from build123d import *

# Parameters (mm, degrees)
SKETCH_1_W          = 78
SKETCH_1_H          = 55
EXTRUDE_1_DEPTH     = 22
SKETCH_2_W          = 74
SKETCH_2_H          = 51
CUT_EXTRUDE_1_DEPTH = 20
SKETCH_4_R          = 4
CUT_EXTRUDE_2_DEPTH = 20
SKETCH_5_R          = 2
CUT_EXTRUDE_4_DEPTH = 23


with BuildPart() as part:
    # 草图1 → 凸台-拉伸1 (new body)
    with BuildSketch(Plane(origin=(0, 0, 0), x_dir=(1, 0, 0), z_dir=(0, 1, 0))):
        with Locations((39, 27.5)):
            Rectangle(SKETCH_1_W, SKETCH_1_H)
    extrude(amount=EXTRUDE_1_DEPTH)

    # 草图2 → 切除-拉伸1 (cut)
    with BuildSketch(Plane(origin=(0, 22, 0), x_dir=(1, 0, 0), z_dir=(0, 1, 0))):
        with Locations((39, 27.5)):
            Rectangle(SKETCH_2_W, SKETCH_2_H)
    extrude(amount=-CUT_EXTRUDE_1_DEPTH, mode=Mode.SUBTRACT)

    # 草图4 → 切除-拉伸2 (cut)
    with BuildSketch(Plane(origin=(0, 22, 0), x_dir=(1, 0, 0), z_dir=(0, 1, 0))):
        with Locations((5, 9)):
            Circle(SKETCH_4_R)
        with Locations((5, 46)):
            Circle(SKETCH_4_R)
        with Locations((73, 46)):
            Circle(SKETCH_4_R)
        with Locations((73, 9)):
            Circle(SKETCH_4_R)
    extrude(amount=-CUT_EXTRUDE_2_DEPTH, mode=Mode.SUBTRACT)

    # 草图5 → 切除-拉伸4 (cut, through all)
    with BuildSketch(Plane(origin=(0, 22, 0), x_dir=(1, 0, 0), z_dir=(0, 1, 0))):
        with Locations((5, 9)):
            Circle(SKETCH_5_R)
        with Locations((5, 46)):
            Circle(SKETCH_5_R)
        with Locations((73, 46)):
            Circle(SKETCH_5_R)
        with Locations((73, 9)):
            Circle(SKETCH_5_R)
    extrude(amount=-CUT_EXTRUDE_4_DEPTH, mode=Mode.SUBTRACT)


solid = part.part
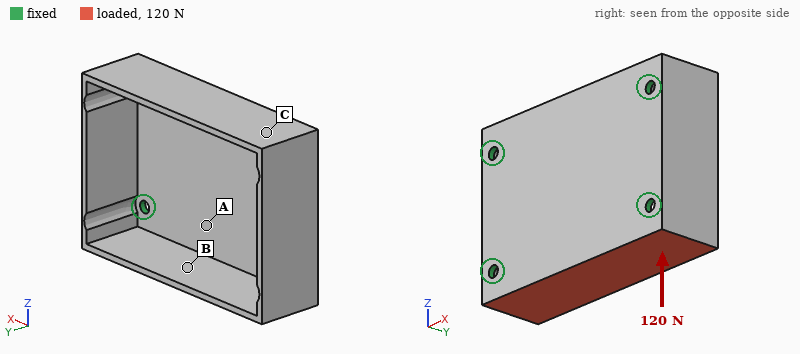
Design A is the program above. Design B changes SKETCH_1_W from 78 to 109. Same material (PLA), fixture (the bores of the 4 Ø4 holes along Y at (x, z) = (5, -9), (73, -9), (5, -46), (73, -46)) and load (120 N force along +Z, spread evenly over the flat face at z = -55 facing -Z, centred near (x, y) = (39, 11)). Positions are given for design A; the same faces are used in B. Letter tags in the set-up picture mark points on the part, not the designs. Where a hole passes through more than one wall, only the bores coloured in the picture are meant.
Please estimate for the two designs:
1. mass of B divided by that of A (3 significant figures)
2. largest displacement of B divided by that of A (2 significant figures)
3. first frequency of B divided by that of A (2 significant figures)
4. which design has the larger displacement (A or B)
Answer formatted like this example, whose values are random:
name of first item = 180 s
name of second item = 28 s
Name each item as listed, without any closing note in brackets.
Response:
mass of B divided by that of A = 3.03
largest displacement of B divided by that of A = 0.58
first frequency of B divided by that of A = 1.1
which design has the larger displacement = A
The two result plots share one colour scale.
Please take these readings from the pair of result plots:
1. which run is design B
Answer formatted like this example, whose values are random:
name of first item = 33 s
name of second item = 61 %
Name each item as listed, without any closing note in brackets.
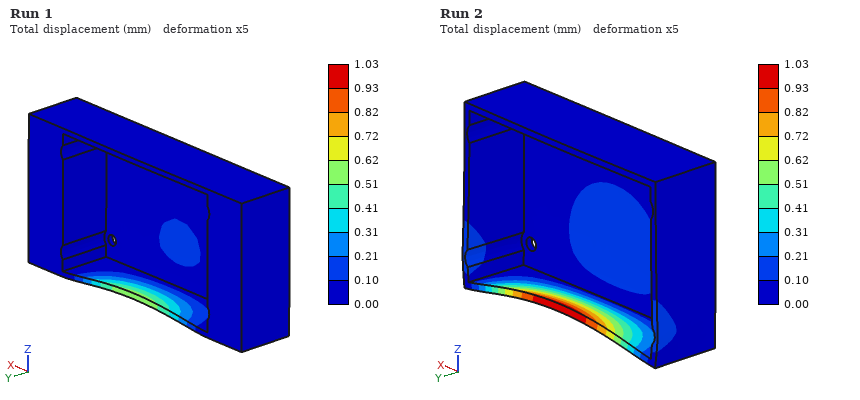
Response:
which run is design B = Run 1
